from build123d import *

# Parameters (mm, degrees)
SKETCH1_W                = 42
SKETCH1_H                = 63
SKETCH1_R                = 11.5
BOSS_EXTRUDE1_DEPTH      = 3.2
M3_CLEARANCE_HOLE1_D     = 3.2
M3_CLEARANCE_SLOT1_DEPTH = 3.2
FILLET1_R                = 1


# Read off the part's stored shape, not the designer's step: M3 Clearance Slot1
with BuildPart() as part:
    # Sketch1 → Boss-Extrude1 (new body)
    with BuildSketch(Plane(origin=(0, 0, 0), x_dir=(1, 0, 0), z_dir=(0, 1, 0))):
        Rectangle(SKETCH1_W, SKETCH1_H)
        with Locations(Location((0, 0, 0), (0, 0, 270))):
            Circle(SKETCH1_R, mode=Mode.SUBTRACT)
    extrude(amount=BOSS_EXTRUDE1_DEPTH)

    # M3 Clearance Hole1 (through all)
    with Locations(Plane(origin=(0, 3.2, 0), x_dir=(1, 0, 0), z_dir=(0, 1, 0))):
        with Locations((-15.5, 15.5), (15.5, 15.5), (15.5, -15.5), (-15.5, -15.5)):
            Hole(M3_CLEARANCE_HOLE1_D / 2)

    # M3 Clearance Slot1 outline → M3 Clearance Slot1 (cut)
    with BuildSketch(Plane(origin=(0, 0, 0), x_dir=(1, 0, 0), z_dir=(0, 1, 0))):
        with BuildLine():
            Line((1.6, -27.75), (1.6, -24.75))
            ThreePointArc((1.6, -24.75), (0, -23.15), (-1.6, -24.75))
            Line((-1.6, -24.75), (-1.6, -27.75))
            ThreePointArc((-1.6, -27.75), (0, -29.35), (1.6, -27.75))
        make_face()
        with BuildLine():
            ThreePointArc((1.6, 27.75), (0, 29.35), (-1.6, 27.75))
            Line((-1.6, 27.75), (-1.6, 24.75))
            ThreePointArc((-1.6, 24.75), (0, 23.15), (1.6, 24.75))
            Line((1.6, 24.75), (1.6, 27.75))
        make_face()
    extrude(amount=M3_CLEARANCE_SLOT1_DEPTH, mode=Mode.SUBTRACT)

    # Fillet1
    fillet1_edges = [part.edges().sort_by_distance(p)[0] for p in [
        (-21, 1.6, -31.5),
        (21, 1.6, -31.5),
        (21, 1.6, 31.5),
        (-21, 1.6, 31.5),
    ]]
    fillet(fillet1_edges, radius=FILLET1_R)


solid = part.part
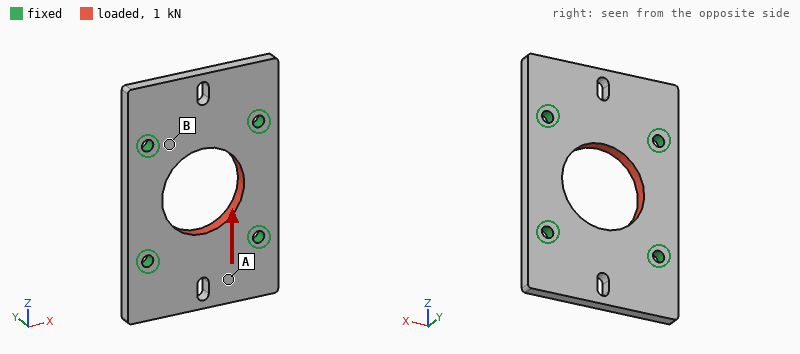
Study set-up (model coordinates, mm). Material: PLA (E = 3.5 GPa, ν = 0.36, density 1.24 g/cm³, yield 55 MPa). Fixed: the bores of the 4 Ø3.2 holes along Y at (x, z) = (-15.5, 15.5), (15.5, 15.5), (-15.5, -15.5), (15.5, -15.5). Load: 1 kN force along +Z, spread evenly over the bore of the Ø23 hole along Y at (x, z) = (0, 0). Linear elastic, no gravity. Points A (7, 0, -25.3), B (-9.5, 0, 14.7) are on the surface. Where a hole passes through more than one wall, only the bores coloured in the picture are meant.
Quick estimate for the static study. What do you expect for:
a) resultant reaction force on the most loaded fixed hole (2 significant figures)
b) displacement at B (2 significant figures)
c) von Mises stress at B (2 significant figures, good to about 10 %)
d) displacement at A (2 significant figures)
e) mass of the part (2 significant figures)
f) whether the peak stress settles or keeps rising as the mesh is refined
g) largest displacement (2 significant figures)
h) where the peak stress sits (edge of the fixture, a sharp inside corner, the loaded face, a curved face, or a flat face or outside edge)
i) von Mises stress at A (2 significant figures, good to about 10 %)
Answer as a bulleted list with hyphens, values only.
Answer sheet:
- 250 N
- 18 µm
- 4.1 MPa
- 21 µm
- 8.6 g
- keeps rising
- 38 µm
- edge of the fixture
- 2.0 MPa
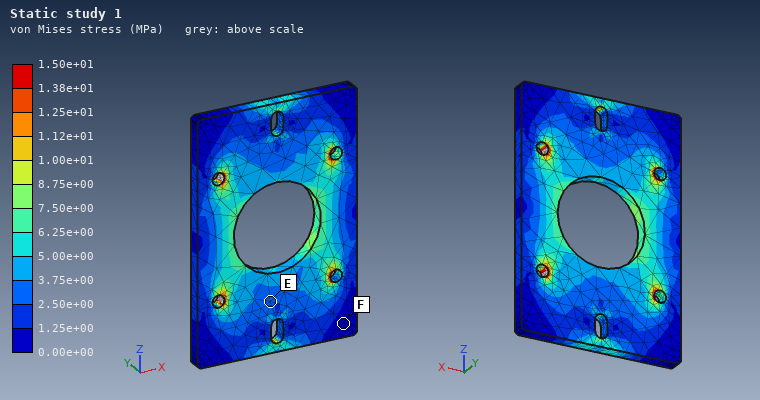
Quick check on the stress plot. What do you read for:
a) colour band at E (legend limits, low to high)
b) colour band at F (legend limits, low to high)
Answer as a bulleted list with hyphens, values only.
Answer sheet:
- 2.50e+00 to 3.75e+00 MPa
- 0.00e+00 to 1.25e+00 MPa
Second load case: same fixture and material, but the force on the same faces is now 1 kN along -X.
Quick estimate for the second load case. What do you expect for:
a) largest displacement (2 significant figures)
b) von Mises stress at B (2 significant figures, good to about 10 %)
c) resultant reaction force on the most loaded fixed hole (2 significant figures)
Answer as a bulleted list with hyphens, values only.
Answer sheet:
- 58 µm
- 7.0 MPa
- 260 N
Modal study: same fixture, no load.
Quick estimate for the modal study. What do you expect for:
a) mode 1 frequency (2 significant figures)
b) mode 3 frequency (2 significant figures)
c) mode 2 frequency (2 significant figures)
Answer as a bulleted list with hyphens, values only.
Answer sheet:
- 2700 Hz
- 4300 Hz
- 2800 Hz
